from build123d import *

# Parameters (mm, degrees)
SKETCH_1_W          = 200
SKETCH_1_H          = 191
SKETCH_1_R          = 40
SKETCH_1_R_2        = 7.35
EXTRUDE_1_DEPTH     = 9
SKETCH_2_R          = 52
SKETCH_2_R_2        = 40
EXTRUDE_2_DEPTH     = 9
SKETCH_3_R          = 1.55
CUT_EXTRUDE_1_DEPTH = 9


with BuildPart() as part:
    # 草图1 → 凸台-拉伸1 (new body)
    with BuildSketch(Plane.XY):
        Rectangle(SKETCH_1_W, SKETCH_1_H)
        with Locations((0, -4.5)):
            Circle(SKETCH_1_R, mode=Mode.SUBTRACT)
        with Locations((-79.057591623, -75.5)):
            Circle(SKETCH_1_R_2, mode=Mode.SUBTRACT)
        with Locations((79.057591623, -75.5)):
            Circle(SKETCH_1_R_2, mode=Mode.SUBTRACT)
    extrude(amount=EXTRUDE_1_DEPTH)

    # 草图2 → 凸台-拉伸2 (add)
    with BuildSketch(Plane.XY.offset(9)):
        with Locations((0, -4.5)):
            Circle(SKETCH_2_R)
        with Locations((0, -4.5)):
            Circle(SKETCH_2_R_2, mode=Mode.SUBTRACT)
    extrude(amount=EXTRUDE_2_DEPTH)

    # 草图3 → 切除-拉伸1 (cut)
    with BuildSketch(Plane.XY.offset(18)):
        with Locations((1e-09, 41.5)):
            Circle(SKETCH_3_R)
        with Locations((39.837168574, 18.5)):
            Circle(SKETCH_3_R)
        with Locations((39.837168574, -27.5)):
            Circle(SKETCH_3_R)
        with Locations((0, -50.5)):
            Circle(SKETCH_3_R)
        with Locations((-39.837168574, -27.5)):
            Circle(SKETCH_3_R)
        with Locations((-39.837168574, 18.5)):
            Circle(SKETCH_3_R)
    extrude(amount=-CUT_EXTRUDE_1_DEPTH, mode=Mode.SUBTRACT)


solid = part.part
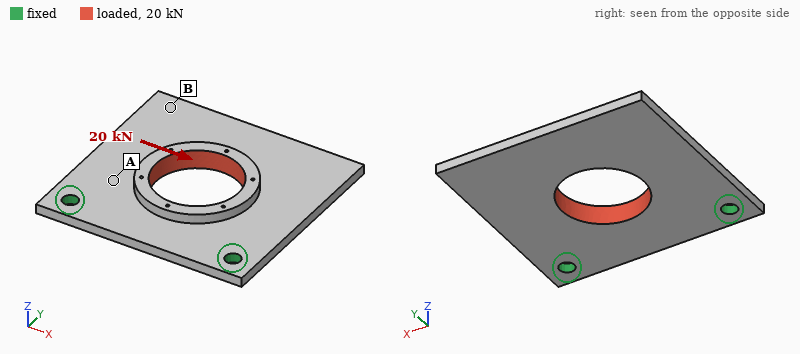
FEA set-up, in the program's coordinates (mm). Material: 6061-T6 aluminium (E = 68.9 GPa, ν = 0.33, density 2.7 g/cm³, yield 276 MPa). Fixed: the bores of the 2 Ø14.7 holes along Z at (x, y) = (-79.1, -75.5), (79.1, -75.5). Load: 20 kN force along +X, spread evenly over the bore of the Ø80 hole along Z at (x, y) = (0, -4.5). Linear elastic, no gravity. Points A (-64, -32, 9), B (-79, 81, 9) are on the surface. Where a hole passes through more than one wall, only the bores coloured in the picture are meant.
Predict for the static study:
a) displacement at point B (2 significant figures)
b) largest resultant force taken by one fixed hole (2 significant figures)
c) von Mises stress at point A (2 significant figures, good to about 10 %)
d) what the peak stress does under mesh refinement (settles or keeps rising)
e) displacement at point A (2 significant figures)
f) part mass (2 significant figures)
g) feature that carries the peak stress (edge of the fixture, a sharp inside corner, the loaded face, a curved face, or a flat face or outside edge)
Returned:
0.14 mm
13 kN
32 MPa
keeps rising
0.045 mm
880 g
edge of the fixture
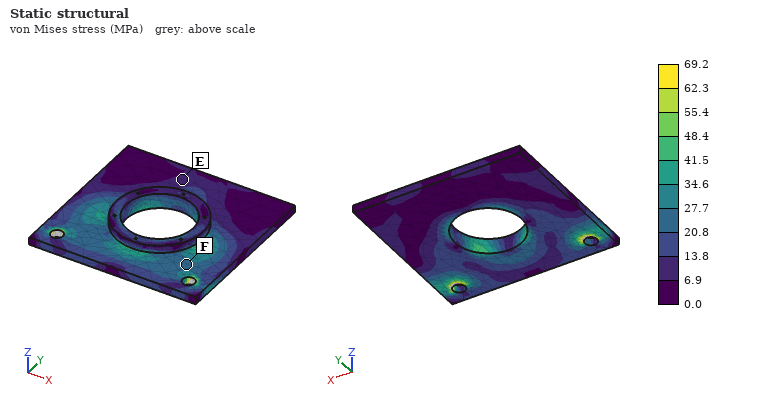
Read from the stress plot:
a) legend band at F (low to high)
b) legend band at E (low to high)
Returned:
20.8 to 27.7 MPa
6.9 to 13.8 MPa
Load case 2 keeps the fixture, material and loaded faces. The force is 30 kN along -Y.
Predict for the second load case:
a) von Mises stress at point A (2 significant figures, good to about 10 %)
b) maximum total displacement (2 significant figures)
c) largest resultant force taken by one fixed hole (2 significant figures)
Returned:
58 MPa
1.6 mm
16 kN
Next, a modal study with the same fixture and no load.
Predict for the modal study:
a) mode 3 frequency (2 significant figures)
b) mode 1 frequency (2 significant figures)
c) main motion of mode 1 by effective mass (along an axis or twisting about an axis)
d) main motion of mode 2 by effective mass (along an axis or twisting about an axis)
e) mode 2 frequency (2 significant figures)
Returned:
1600 Hz
240 Hz
along Z
twisting about Y
610 Hz
